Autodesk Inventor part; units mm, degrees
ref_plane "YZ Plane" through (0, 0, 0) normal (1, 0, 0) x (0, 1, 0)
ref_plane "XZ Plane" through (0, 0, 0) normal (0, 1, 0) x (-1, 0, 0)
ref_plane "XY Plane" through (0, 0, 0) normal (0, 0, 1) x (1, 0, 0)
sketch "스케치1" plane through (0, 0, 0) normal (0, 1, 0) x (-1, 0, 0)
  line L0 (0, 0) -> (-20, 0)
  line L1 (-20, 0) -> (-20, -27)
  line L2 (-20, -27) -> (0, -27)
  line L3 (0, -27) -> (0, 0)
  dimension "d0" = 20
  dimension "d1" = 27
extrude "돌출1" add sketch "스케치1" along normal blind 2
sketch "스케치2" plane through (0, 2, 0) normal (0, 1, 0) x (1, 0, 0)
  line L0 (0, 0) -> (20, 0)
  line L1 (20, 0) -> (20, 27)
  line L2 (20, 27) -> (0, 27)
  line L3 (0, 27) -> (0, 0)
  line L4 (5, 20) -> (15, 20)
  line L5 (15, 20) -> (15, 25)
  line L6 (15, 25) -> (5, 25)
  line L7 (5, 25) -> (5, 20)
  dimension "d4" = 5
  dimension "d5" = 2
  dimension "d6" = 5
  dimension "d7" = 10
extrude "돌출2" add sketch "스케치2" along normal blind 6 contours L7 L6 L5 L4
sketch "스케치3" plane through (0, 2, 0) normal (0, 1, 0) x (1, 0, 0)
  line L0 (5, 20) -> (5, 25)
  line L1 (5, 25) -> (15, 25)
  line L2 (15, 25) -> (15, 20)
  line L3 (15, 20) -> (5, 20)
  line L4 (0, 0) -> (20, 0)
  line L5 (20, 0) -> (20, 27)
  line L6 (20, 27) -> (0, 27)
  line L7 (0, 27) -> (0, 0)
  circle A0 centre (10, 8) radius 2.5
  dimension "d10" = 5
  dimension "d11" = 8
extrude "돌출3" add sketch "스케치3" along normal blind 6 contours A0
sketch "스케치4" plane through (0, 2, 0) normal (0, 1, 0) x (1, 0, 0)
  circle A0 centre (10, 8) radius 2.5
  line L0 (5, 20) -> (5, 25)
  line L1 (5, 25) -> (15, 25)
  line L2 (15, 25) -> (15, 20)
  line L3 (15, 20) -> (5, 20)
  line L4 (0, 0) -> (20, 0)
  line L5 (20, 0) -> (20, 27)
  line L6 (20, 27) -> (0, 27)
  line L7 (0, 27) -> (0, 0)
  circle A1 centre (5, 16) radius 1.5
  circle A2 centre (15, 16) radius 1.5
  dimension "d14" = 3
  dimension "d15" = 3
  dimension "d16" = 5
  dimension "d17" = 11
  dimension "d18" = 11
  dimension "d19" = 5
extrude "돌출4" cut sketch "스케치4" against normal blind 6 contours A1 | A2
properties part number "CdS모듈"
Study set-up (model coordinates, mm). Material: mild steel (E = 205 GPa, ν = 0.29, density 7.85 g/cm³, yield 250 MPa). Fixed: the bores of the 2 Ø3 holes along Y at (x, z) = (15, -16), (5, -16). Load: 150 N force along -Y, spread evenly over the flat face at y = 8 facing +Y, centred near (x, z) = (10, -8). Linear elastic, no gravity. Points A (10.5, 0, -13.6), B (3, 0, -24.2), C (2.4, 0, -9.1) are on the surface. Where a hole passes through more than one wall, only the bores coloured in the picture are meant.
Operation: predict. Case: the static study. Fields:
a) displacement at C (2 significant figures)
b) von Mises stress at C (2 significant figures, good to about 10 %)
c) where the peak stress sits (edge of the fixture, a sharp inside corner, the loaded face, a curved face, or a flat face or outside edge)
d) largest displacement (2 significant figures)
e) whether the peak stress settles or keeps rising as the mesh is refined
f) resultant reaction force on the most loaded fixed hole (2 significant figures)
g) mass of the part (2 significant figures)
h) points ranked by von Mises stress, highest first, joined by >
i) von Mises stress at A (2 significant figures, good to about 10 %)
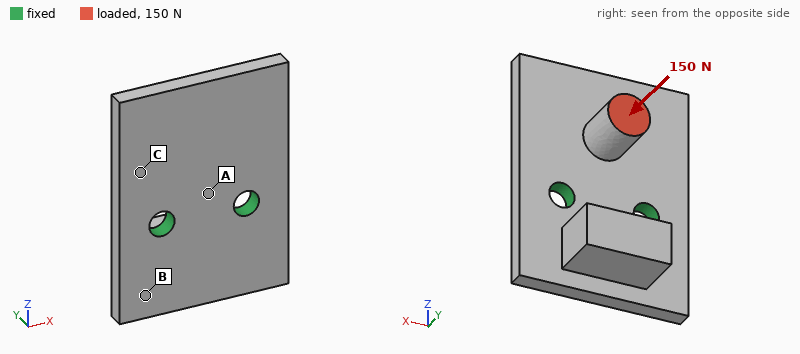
5.4 µm
21 MPa
edge of the fixture
21 µm
keeps rising
75 N
12 g
A > C > B
49 MPa
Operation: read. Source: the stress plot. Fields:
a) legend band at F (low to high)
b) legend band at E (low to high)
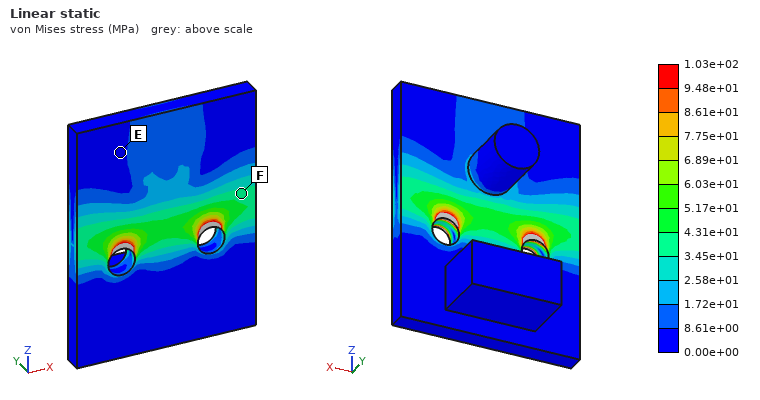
3.45e+01 to 4.31e+01 MPa
0.00e+00 to 8.61e+00 MPa
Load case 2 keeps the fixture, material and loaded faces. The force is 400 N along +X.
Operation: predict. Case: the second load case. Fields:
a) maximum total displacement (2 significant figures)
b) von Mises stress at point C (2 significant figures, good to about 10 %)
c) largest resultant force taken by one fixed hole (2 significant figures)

29 µm
38 MPa
410 N
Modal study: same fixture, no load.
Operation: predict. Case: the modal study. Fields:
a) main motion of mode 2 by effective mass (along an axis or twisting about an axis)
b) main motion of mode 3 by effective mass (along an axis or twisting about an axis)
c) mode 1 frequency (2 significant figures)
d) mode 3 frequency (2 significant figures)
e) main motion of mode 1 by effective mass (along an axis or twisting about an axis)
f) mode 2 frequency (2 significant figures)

along Y
twisting about Z
6600 Hz
14 kHz
along Y
10 kHz
